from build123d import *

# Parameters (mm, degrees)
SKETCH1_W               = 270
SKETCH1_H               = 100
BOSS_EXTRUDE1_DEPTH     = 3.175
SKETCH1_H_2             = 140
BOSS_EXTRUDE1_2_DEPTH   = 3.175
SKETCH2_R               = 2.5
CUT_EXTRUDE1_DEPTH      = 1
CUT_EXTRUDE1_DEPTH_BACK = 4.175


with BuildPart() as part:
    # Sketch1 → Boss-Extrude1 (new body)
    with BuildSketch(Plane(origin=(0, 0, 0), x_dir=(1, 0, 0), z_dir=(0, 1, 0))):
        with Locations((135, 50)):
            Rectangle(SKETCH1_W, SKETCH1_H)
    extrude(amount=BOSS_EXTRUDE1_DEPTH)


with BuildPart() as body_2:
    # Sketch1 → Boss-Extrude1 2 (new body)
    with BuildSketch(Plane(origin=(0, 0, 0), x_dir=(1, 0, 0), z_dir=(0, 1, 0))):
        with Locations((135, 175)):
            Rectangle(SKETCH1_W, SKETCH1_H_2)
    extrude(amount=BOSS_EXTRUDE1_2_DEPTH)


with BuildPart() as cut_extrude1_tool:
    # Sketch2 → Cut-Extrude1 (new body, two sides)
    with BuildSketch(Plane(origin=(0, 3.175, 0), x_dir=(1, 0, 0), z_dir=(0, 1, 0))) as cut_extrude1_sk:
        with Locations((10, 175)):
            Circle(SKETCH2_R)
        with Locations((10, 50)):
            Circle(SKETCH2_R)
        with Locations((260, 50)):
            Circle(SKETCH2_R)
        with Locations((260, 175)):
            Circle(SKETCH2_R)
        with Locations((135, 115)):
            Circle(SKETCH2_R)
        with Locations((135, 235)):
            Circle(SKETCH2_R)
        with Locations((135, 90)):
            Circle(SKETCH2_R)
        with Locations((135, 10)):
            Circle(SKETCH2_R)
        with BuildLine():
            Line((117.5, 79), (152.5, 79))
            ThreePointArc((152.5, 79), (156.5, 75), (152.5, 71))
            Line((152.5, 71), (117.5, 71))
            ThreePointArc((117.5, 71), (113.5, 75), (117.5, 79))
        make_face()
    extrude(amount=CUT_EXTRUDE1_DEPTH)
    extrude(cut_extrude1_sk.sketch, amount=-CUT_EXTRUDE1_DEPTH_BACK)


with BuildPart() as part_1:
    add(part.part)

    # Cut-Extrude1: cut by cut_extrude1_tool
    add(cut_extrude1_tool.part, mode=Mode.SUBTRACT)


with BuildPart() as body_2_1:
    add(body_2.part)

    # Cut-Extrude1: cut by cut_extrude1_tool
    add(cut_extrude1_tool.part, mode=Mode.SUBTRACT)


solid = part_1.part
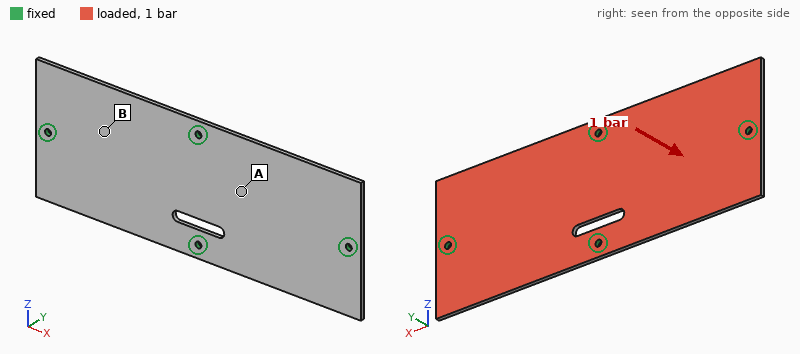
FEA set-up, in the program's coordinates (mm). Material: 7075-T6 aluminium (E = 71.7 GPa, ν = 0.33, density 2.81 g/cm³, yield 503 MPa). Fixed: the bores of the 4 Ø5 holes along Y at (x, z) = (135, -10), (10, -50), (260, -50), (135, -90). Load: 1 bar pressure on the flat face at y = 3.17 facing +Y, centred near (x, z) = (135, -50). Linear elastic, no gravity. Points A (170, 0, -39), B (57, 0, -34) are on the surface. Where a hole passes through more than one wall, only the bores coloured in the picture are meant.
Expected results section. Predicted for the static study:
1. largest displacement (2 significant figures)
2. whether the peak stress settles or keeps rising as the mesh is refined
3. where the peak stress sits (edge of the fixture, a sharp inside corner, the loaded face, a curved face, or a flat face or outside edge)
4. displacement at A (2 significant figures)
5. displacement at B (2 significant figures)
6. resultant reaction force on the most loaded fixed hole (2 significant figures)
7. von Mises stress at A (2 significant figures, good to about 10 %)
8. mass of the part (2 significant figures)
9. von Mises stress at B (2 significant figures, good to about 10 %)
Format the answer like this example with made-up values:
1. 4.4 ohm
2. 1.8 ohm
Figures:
1. 0.66 mm
2. keeps rising
3. edge of the fixture
4. 0.35 mm
5. 0.45 mm
6. 710 N
7. 18 MPa
8. 240 g
9. 44 MPa
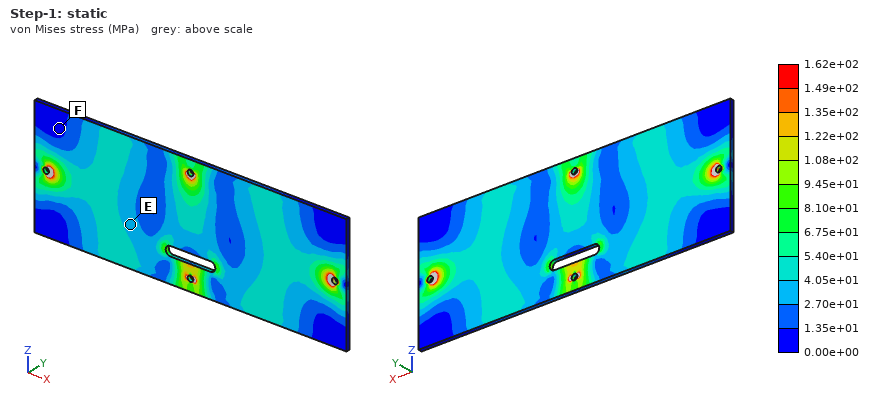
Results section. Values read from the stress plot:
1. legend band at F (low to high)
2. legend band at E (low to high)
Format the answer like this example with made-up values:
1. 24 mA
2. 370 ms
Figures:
1. 0.00e+00 to 1.35e+01 MPa
2. 2.70e+01 to 4.05e+01 MPa
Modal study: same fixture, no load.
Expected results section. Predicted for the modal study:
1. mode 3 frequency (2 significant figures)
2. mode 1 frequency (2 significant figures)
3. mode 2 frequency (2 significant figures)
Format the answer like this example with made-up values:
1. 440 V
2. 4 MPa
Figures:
1. 790 Hz
2. 780 Hz
3. 790 Hz
